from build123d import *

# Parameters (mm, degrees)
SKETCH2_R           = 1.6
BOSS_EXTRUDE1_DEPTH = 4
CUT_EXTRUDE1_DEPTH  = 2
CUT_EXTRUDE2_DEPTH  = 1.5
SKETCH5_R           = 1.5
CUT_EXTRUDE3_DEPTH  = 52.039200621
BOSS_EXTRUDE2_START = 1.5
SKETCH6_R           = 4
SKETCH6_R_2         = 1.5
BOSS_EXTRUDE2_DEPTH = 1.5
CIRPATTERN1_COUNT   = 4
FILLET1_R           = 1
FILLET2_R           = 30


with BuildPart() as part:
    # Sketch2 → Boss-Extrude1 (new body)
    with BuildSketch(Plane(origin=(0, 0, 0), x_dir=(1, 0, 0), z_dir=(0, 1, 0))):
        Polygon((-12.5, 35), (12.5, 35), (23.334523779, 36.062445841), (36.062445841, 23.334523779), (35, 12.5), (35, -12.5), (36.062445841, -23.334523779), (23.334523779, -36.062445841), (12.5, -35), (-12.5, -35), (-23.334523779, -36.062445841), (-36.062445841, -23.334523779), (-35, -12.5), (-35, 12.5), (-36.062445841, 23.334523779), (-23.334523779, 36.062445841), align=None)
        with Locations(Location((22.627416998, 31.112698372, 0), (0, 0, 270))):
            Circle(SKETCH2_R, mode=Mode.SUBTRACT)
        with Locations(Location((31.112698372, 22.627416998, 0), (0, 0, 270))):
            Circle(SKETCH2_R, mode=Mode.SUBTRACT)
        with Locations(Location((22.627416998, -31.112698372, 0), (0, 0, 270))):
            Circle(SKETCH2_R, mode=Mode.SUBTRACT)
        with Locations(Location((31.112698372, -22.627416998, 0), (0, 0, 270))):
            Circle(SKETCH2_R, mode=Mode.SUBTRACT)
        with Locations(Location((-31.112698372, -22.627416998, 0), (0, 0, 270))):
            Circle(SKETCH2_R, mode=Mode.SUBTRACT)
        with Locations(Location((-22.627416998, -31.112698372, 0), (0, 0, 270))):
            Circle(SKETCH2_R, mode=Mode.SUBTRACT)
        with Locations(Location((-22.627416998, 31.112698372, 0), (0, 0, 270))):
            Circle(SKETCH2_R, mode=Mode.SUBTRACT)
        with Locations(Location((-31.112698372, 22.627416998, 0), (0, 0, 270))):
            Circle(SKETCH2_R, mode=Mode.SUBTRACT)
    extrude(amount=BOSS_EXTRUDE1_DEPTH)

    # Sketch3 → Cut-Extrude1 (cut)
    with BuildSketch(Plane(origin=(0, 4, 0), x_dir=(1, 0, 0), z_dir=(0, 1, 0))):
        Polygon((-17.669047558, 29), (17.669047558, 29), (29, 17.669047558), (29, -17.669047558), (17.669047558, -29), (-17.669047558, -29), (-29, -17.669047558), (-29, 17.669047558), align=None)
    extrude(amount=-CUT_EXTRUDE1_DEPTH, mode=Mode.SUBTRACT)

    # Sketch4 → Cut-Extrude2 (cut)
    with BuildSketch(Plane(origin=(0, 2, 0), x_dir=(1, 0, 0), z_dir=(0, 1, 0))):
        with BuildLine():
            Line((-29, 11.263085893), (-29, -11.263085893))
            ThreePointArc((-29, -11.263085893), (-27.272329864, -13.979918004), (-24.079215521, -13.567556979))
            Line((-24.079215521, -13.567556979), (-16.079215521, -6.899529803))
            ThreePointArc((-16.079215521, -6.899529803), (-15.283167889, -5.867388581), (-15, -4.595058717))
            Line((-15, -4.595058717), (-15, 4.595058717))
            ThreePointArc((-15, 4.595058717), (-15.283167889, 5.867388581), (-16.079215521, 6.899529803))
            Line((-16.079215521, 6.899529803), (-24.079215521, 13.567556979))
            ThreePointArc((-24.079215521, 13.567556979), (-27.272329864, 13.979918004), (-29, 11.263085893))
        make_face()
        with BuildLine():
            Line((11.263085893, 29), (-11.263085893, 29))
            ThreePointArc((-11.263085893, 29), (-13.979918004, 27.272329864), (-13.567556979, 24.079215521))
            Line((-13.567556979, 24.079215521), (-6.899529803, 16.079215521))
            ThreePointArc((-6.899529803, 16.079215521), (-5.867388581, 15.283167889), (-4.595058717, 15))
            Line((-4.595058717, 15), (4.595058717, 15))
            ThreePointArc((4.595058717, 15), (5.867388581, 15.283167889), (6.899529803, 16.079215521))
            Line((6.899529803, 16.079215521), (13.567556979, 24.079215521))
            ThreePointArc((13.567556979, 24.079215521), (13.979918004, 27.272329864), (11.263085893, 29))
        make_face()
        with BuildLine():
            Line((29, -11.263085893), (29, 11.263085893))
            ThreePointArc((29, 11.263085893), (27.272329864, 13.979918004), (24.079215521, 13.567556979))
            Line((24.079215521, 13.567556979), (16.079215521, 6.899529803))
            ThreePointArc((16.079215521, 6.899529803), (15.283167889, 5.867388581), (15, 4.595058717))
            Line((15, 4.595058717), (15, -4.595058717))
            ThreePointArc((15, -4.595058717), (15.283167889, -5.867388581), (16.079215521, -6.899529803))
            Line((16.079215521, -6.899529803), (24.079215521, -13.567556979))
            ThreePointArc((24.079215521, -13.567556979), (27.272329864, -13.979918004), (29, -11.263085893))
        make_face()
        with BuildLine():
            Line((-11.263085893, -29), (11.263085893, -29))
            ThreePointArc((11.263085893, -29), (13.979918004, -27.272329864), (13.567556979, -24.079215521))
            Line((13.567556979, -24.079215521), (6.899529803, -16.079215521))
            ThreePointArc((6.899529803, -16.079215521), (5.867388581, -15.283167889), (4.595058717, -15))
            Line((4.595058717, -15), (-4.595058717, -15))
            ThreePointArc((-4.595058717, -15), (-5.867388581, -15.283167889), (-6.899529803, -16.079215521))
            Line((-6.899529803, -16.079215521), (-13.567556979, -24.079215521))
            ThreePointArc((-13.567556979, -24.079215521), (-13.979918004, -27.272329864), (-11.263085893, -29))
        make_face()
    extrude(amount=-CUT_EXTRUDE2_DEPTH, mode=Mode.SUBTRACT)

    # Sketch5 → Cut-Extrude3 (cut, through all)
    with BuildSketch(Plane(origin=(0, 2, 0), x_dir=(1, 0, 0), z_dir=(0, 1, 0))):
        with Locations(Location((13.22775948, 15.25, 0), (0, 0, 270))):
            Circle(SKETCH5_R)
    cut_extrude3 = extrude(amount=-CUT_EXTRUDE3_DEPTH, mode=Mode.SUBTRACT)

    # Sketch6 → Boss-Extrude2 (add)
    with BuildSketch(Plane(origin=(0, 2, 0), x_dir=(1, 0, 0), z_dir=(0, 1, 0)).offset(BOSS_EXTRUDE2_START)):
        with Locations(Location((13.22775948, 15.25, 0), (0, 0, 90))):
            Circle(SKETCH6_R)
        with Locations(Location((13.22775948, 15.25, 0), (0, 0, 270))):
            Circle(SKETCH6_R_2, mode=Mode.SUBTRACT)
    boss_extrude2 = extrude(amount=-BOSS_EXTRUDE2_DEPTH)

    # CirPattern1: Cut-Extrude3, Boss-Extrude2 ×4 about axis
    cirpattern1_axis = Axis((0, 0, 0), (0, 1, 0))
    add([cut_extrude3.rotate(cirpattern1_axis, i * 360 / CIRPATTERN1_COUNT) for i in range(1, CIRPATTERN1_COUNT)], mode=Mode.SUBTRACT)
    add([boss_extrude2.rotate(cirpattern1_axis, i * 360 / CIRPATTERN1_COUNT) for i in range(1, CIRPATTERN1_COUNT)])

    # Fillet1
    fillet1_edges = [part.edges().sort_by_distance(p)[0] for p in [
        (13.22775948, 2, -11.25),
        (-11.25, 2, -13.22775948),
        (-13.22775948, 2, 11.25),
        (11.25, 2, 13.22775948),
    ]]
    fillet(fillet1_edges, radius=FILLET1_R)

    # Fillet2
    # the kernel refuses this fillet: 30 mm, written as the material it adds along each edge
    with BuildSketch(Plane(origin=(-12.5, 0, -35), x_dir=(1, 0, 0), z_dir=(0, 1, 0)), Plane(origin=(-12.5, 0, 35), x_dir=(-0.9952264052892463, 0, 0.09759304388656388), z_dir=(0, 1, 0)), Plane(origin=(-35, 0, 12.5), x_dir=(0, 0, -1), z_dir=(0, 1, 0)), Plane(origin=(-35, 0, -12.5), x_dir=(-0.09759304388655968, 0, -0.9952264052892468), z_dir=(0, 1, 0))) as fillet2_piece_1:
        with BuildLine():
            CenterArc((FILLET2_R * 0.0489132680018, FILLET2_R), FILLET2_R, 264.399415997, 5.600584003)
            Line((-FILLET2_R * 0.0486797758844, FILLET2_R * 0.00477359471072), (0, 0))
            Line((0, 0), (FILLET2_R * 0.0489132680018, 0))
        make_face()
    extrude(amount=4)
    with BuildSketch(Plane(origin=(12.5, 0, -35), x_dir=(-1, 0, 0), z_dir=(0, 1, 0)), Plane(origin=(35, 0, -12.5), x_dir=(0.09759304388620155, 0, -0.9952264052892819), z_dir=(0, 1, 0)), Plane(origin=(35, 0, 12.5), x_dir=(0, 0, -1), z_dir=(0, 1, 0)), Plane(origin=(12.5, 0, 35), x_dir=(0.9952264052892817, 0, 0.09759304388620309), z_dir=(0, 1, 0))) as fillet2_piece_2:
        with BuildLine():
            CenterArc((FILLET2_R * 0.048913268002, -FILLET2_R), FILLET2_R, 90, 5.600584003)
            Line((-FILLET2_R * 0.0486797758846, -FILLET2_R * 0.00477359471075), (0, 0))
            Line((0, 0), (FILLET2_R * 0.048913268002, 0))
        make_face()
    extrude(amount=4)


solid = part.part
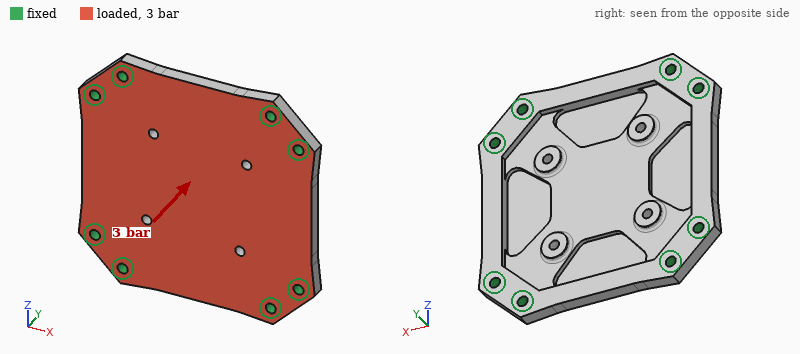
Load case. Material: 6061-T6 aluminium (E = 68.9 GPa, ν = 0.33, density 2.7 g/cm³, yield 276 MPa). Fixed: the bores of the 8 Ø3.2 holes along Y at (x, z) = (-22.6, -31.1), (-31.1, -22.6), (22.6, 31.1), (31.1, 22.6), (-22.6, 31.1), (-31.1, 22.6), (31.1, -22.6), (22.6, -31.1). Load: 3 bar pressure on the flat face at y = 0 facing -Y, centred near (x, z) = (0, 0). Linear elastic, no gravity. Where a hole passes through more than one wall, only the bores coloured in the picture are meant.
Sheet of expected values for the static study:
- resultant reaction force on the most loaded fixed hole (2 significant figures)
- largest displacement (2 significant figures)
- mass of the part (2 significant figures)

210 N
0.22 mm
29 g
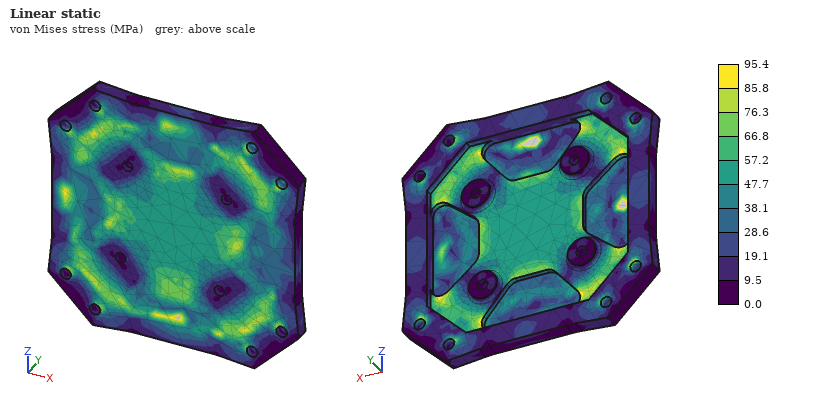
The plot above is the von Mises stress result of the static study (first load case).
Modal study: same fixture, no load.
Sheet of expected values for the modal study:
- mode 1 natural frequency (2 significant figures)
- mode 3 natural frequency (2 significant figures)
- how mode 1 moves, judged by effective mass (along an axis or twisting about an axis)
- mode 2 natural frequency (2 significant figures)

3300 Hz
7200 Hz
along Y
7200 Hz
